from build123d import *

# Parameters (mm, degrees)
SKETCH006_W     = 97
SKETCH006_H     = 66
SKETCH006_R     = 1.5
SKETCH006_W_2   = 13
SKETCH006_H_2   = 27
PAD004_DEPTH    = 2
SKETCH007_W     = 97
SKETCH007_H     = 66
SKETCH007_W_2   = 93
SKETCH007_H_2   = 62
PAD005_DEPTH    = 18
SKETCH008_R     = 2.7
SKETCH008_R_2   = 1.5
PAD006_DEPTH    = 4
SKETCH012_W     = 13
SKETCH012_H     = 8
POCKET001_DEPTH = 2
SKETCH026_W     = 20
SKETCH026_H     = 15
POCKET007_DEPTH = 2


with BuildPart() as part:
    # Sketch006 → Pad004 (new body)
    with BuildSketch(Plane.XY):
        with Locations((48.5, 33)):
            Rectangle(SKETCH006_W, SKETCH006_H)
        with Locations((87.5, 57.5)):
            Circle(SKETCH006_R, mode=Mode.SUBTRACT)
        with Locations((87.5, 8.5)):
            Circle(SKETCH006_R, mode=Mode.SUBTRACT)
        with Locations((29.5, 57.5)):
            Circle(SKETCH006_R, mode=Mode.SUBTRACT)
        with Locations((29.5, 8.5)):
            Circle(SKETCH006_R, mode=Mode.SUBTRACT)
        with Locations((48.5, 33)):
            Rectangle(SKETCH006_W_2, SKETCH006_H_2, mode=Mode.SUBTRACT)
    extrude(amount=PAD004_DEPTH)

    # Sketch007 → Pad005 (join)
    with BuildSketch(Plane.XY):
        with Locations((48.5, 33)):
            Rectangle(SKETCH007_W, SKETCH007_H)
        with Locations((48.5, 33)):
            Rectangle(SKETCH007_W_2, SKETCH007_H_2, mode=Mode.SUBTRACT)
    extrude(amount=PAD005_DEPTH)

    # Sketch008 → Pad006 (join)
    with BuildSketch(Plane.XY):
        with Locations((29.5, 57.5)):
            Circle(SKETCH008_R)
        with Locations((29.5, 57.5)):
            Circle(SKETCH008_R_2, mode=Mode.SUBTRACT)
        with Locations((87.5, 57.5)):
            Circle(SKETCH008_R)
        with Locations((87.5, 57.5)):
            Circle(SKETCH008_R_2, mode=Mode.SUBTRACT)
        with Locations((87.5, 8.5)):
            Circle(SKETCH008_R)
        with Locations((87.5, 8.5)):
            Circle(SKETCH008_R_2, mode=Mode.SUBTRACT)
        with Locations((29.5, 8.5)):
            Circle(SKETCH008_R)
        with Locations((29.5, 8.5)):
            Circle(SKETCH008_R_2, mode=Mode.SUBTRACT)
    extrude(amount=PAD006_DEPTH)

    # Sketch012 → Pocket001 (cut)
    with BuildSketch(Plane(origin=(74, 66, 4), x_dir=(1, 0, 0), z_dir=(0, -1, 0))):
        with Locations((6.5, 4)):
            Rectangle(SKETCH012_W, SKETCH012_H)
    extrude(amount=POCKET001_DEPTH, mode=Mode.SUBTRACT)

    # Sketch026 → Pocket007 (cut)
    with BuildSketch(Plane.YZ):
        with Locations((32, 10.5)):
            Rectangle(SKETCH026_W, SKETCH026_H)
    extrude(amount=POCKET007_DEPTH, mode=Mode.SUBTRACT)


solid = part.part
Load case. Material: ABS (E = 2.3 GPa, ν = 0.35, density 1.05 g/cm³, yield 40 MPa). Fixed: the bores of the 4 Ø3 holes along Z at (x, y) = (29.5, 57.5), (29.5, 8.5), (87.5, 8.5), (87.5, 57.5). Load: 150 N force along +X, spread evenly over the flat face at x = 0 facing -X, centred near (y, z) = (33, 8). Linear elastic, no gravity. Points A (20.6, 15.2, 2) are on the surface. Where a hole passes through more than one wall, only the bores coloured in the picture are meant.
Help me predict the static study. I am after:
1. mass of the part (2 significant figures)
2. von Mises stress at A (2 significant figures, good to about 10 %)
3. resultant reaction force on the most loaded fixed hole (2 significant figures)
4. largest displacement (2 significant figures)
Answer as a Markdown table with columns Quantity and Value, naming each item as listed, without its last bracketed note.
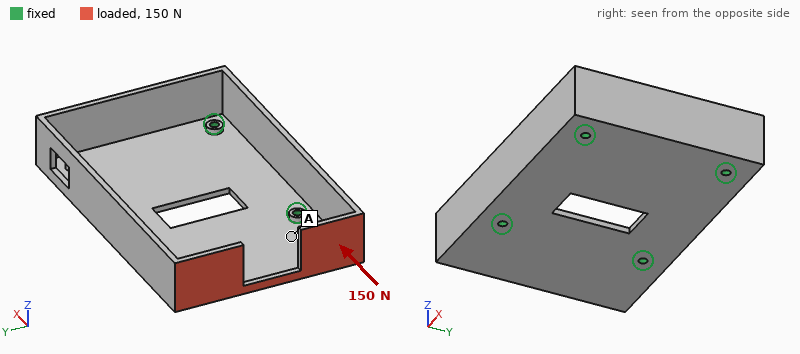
| Quantity | Value |
|---|---|
| mass of the part | 23 g |
| von Mises stress at A | 1.9 MPa |
| resultant reaction force on the most loaded fixed hole | 52 N |
| largest displacement | 1.2 mm |
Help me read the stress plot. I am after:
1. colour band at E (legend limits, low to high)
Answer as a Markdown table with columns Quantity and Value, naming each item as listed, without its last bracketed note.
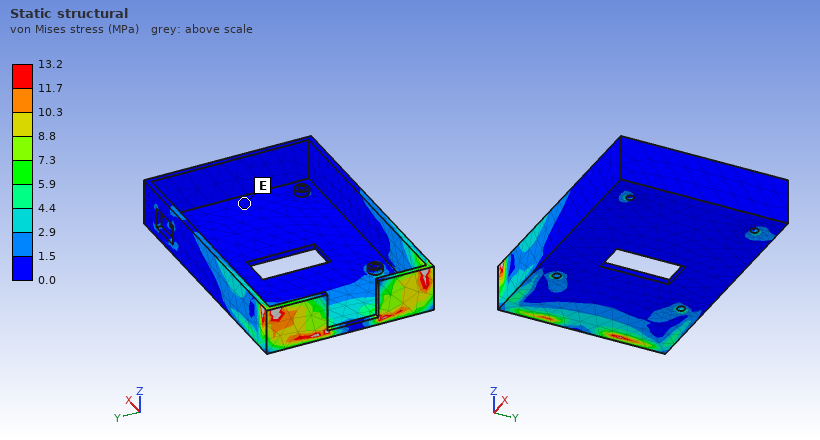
| Quantity | Value |
|---|---|
| colour band at E | 0.0 to 1.5 MPa |
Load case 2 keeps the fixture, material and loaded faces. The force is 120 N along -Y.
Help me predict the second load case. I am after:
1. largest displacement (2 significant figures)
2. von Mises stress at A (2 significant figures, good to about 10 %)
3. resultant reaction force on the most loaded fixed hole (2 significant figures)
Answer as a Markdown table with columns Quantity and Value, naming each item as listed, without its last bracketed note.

| Quantity | Value |
|---|---|
| largest displacement | 0.44 mm |
| von Mises stress at A | 3.6 MPa |
| resultant reaction force on the most loaded fixed hole | 98 N |
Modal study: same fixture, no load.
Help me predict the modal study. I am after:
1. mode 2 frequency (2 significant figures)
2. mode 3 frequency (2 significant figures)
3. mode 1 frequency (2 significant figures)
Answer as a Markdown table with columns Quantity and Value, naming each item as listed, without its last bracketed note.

| Quantity | Value |
|---|---|
| mode 2 frequency | 830 Hz |
| mode 3 frequency | 1000 Hz |
| mode 1 frequency | 620 Hz |
